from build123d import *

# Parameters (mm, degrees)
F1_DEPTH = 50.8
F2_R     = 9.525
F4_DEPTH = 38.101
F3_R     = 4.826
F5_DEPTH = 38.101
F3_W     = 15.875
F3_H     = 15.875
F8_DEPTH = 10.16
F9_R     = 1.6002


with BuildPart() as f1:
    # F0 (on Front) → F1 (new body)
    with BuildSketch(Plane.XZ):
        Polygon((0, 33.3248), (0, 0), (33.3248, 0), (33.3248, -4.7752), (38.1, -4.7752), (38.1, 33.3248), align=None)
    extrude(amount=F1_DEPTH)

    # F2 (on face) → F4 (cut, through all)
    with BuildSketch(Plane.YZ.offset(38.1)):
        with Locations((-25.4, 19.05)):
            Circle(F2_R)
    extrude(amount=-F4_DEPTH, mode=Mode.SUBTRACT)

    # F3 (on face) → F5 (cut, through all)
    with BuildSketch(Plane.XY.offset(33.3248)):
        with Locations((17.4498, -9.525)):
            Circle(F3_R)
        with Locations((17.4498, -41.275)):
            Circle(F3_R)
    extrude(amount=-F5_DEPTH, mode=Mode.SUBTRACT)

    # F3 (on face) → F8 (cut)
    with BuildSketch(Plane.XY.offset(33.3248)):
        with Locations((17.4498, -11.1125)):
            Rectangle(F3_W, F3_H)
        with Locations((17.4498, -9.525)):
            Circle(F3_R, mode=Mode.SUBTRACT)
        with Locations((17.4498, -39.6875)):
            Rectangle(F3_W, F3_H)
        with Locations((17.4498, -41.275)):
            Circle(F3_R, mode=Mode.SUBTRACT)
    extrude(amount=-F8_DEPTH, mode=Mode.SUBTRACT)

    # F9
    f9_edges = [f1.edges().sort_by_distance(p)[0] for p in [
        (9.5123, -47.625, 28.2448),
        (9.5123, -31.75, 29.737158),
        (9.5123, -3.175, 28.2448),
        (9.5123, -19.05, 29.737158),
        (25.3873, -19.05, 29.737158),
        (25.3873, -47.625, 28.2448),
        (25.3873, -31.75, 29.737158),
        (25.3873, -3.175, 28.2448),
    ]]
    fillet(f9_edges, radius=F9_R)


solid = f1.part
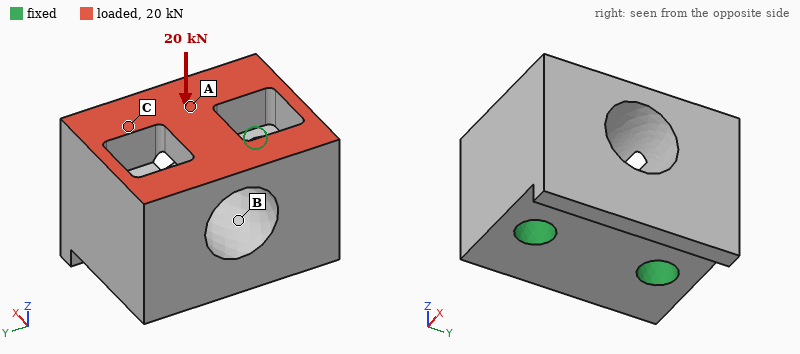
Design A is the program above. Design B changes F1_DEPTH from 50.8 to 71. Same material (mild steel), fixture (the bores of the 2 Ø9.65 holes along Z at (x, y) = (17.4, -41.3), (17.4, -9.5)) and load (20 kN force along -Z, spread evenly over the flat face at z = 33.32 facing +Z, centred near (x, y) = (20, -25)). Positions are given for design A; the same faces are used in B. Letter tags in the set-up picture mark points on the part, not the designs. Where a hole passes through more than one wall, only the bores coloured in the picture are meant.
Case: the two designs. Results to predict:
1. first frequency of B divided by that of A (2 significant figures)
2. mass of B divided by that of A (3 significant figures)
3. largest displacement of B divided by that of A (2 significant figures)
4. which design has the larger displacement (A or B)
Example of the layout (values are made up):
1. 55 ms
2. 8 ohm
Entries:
1. 0.62
2. 1.56
3. 0.68
4. A
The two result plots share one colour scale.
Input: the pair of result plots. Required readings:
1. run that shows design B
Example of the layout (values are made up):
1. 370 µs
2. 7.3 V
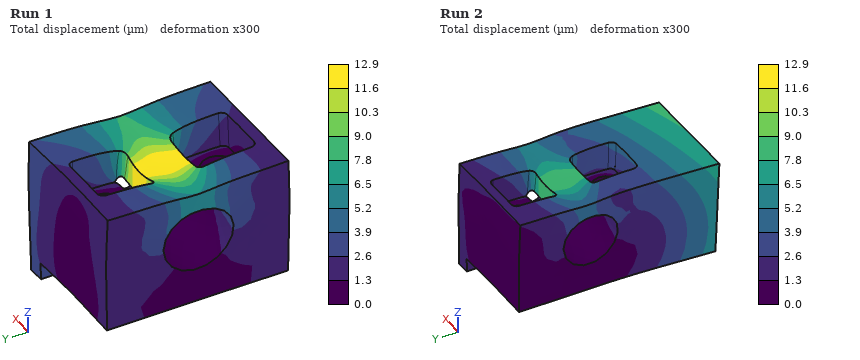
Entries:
1. Run 2
